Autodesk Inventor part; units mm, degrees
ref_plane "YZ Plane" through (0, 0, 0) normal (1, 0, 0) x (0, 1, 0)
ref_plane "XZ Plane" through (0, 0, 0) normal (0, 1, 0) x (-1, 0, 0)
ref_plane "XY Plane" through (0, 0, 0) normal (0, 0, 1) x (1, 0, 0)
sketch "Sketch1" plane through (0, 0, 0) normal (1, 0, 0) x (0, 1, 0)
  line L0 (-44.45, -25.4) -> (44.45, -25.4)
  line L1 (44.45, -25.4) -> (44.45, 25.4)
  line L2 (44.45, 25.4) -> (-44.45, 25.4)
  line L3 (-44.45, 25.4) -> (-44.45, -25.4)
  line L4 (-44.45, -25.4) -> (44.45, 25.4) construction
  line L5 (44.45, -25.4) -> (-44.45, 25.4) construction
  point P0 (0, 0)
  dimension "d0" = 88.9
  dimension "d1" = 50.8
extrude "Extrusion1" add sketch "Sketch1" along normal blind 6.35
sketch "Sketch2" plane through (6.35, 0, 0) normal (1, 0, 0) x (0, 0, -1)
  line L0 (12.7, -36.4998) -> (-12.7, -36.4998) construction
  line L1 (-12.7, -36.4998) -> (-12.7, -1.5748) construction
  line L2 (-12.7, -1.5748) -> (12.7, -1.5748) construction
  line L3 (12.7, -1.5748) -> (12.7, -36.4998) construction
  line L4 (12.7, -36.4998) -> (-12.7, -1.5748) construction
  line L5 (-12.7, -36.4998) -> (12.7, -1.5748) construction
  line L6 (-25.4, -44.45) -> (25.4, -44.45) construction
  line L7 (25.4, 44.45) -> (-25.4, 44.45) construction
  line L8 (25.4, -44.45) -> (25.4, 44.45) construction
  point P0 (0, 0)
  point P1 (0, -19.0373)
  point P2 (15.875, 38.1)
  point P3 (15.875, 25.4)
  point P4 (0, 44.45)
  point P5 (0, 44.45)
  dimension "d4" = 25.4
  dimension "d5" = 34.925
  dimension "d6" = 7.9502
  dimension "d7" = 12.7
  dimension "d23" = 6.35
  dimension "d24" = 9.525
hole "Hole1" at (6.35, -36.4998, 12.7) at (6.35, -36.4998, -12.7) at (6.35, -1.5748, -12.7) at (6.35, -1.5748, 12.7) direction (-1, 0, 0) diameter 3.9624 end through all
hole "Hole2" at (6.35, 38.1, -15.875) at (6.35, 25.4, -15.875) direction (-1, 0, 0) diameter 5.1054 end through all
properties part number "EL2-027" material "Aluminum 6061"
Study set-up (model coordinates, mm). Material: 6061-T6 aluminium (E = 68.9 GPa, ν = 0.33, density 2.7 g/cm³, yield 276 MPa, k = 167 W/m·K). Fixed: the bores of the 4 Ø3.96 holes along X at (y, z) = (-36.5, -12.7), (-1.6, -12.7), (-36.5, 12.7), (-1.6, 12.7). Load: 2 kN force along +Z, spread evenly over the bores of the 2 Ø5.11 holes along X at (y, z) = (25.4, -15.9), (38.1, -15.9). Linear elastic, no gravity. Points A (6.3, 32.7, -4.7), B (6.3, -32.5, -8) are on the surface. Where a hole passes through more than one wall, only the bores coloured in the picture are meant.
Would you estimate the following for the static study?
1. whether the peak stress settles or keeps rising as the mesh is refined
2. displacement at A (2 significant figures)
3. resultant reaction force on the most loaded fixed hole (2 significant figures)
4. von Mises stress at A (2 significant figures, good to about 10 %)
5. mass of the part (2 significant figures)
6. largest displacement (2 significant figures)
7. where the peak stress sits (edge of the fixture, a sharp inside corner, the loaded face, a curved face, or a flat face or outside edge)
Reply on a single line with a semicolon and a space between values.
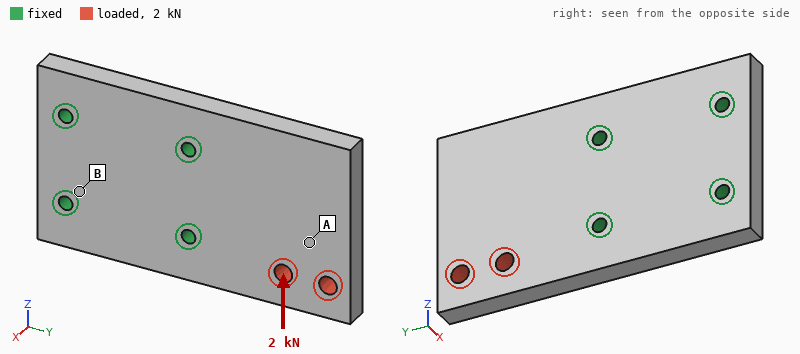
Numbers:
keeps rising; 19 µm; 2.0 kN; 11 MPa; 76 g; 28 µm; edge of the fixture
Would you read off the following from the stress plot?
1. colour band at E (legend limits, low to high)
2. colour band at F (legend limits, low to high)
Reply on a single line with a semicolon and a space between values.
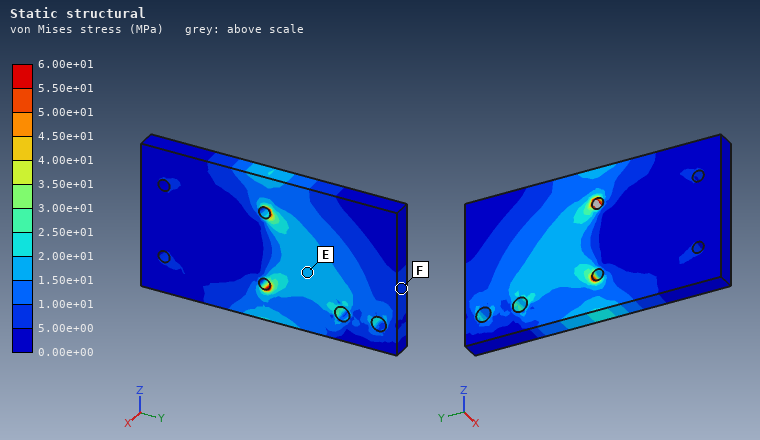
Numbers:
1.50e+01 to 2.00e+01 MPa; 5.00e+00 to 1.00e+01 MPa
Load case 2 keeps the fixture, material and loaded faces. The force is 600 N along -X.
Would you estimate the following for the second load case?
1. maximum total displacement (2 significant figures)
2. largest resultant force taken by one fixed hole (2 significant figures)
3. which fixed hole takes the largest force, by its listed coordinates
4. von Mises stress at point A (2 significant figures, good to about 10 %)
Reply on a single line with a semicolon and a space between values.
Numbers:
0.23 mm; 710 N; (-1.6, -12.7); 18 MPa
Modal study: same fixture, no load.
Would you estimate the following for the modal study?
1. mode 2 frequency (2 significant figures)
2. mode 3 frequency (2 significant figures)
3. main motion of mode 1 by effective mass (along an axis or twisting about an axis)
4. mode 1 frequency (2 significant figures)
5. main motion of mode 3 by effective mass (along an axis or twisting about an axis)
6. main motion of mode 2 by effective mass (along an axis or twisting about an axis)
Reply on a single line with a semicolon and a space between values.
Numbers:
5000 Hz; 10 kHz; along X; 2400 Hz; along Z; twisting about Y
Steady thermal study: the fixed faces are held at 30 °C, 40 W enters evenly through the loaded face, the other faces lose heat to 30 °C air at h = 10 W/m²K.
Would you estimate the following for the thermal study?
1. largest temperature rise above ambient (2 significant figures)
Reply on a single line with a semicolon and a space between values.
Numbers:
40 K
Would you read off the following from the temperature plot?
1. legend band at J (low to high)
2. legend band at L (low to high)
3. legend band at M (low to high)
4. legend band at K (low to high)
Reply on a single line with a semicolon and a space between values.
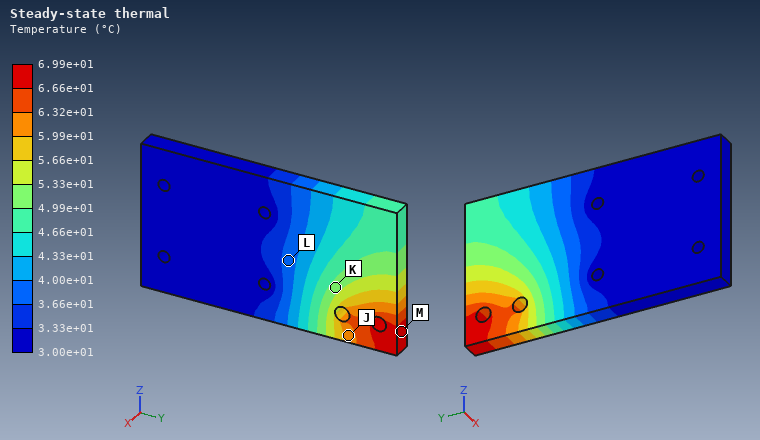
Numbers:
5.99e+01 to 6.32e+01 °C; 3.66e+01 to 4.00e+01 °C; 6.66e+01 to 6.99e+01 °C; 4.99e+01 to 5.33e+01 °C
